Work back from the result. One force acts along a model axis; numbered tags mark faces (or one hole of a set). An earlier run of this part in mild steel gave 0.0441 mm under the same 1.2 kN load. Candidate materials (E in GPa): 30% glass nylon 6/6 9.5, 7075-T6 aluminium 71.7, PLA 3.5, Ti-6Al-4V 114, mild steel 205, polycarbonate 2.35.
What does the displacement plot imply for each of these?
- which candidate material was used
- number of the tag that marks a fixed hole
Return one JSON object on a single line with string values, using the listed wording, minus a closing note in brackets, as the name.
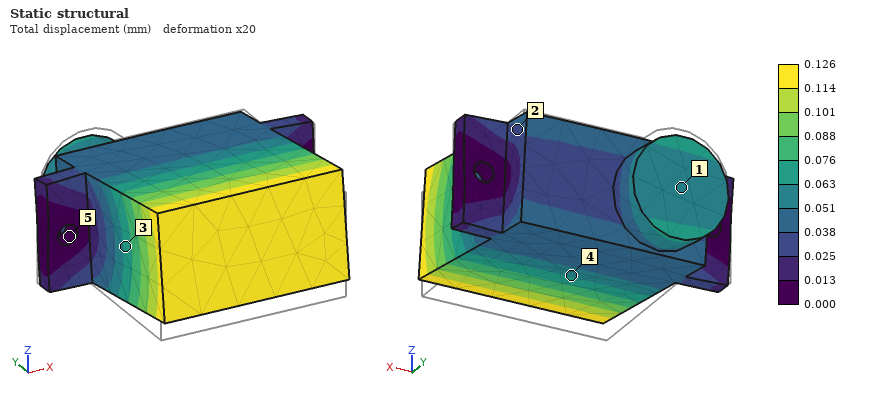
{"which candidate material was used": "7075-T6 aluminium", "number of the tag that marks a fixed hole": "5"}
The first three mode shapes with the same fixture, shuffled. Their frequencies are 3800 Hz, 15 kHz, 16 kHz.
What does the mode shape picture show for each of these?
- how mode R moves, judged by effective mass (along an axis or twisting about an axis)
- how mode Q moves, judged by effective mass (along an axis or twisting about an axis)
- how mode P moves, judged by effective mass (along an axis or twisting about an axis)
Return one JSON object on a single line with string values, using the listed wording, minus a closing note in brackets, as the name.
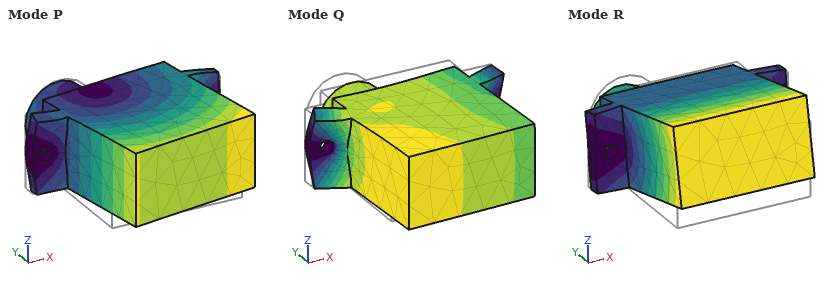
{"how mode R moves, judged by effective mass": "along Z", "how mode Q moves, judged by effective mass": "along Y", "how mode P moves, judged by effective mass": "along X"}
